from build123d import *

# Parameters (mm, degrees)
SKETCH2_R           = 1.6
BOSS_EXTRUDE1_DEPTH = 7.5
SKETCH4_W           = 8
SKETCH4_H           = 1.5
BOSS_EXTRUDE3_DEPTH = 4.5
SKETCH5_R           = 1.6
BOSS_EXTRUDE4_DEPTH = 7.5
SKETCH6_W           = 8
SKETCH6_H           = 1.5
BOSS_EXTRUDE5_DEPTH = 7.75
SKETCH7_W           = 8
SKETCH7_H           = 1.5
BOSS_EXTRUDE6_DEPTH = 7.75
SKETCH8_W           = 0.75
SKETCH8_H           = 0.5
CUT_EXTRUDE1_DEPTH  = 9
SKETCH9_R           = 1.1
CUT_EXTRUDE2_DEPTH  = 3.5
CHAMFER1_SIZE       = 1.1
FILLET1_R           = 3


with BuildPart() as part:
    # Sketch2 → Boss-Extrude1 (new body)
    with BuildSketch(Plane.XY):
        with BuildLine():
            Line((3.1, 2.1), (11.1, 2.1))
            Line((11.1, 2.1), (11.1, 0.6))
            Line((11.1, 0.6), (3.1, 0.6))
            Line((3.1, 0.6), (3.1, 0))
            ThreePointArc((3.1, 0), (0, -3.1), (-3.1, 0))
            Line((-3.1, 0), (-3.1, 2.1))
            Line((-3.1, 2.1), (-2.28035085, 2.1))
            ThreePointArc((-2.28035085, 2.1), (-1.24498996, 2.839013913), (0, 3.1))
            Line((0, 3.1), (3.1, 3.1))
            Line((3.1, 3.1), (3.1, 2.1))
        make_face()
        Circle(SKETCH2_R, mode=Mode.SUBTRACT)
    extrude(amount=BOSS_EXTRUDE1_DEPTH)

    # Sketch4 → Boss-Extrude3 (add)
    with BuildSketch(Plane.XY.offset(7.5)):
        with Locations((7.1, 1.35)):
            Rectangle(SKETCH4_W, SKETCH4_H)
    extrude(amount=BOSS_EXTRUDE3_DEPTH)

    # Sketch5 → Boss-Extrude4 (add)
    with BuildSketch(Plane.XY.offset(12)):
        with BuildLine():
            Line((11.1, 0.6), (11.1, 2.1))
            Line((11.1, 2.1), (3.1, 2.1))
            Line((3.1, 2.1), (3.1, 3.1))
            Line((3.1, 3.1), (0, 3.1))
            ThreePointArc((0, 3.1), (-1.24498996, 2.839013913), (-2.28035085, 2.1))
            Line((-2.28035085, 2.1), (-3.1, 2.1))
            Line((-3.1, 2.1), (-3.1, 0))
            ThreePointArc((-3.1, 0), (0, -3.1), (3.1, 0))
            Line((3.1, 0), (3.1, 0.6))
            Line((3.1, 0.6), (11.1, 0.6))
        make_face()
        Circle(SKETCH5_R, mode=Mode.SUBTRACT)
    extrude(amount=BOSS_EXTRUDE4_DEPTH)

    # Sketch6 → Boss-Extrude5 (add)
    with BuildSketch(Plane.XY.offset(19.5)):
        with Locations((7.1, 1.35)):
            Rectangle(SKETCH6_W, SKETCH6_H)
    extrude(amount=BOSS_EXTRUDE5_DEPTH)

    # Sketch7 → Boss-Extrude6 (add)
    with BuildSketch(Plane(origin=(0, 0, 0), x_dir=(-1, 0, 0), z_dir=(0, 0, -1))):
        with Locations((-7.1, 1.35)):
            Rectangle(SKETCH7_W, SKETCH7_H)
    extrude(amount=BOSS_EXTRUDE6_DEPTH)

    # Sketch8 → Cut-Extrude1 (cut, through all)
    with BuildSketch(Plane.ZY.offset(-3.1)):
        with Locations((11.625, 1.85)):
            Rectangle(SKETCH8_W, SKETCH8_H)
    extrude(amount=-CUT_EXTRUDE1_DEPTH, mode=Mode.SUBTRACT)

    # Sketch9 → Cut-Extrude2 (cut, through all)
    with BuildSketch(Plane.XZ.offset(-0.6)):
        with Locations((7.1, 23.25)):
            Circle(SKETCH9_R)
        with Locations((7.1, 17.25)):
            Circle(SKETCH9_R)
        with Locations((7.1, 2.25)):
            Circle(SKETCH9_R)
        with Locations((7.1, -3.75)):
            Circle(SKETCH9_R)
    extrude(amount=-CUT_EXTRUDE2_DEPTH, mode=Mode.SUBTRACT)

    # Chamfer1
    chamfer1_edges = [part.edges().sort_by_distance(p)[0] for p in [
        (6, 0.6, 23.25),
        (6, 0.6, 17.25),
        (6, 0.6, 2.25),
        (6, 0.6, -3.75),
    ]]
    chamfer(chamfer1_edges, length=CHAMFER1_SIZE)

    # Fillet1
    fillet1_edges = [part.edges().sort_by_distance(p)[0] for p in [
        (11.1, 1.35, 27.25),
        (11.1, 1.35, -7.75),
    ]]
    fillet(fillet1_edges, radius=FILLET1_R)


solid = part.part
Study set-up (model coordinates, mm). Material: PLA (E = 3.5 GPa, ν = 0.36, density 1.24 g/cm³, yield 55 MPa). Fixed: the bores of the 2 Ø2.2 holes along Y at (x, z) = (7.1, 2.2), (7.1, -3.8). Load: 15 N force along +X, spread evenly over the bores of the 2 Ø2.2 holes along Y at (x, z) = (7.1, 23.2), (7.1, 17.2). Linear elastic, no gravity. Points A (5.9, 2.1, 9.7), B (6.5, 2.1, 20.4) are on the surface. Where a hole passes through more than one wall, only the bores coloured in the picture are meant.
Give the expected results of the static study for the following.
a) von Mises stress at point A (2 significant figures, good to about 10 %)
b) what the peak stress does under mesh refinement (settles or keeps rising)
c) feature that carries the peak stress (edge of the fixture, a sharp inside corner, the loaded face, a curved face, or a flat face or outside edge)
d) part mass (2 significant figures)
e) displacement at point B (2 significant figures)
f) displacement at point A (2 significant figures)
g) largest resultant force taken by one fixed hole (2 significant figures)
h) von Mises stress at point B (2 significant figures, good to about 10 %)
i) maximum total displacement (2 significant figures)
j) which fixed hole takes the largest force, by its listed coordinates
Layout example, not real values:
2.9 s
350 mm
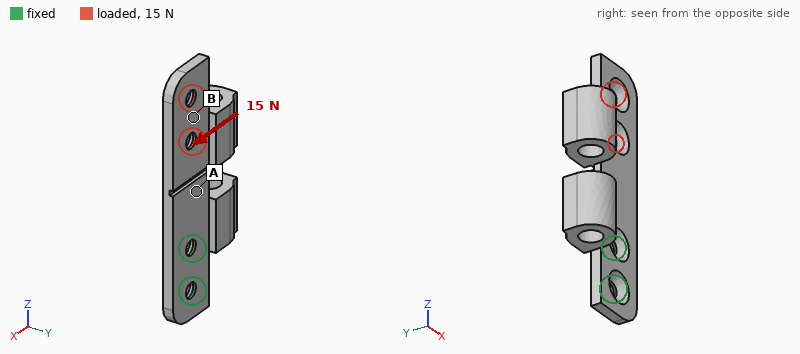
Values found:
8.0 MPa
keeps rising
edge of the fixture
0.91 g
0.22 mm
0.065 mm
46 N
3.8 MPa
0.33 mm
(7.1, 2.2)
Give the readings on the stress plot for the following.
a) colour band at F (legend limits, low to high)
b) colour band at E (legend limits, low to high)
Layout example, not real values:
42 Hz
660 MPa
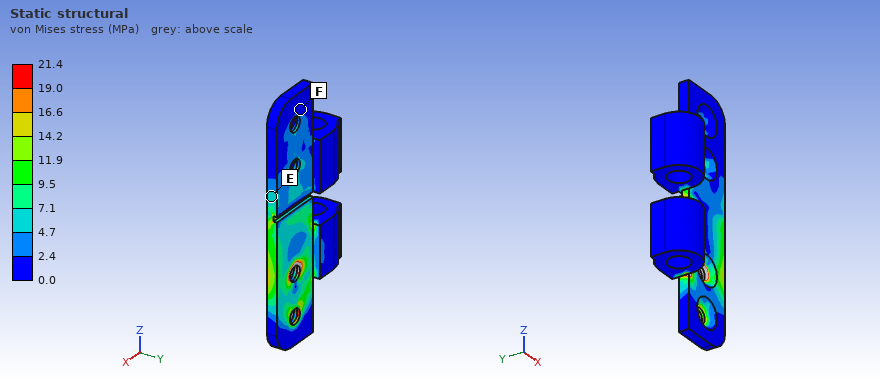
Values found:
0.0 to 2.4 MPa
4.7 to 7.1 MPa
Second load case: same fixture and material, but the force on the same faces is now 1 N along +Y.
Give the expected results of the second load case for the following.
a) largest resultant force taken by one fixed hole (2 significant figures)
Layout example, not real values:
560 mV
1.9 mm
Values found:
5.1 N
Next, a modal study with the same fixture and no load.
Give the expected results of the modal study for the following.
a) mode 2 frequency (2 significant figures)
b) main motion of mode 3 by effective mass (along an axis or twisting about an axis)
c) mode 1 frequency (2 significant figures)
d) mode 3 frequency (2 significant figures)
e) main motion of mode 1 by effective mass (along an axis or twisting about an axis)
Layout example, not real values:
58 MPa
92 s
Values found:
1200 Hz
along X
560 Hz
2200 Hz
along Y
